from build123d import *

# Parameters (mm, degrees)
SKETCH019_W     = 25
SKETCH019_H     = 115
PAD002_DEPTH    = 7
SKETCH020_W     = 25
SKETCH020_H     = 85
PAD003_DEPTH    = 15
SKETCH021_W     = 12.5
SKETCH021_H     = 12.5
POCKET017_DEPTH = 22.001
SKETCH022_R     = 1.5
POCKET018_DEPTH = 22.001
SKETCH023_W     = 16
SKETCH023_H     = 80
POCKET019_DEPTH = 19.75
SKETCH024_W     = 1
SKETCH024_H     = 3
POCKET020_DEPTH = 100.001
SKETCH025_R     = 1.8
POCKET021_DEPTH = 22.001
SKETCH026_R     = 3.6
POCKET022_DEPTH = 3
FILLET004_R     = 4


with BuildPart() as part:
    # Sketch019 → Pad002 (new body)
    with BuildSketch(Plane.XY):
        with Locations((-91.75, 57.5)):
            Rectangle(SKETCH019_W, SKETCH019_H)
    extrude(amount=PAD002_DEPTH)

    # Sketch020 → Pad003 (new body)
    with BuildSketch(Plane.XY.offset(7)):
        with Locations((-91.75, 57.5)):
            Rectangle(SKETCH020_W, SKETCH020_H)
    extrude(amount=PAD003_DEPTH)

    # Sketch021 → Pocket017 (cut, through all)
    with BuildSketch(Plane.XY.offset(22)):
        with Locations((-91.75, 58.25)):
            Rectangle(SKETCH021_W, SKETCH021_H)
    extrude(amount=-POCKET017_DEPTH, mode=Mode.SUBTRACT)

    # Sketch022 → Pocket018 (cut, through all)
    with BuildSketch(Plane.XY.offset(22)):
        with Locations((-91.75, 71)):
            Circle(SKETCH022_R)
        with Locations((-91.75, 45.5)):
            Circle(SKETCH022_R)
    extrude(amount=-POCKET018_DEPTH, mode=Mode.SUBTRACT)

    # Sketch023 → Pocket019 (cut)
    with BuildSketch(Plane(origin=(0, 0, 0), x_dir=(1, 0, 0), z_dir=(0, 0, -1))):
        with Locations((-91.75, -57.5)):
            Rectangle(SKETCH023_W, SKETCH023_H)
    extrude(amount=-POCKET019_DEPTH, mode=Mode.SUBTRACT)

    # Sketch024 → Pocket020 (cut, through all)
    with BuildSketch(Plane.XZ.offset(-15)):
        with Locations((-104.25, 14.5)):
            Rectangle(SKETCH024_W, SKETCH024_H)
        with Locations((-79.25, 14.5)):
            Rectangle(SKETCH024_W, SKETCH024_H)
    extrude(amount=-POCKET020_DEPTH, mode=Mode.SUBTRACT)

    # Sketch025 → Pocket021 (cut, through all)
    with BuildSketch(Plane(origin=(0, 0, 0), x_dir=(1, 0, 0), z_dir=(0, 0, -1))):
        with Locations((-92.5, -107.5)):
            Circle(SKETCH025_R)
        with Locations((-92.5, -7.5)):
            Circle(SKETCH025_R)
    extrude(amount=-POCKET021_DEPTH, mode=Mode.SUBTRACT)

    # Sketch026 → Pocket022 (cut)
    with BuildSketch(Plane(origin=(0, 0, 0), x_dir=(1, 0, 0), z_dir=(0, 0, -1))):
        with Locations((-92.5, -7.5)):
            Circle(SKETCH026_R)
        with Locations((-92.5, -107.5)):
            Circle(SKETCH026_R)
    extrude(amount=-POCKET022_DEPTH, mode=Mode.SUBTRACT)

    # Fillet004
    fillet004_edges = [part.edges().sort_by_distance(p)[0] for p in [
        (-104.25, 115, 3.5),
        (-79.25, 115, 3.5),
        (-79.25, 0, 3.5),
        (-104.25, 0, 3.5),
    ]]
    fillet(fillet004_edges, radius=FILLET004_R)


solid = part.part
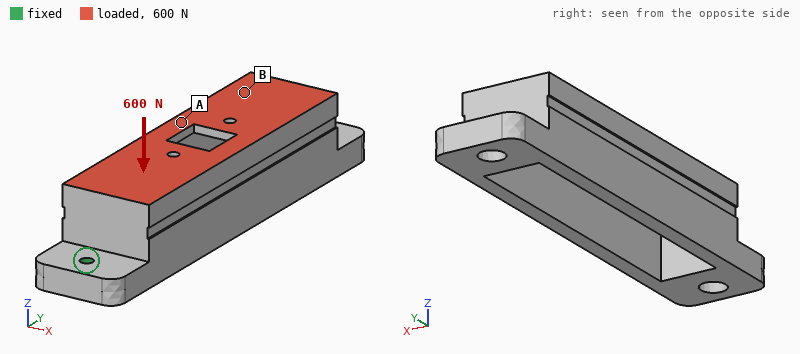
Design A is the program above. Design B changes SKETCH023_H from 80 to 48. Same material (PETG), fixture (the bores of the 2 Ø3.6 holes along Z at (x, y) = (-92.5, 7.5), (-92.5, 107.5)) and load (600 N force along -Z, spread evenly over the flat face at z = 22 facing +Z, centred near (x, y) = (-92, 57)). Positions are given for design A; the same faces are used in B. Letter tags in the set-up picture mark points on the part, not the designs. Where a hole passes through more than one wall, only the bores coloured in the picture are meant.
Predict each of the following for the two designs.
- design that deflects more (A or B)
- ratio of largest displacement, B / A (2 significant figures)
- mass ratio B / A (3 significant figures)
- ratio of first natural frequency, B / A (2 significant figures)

A
0.77
1.39
0.95
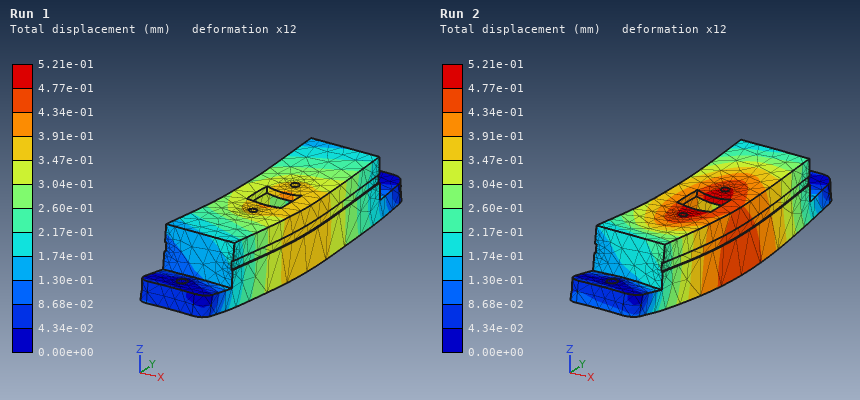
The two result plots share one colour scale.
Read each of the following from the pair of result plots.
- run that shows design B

Run 1
